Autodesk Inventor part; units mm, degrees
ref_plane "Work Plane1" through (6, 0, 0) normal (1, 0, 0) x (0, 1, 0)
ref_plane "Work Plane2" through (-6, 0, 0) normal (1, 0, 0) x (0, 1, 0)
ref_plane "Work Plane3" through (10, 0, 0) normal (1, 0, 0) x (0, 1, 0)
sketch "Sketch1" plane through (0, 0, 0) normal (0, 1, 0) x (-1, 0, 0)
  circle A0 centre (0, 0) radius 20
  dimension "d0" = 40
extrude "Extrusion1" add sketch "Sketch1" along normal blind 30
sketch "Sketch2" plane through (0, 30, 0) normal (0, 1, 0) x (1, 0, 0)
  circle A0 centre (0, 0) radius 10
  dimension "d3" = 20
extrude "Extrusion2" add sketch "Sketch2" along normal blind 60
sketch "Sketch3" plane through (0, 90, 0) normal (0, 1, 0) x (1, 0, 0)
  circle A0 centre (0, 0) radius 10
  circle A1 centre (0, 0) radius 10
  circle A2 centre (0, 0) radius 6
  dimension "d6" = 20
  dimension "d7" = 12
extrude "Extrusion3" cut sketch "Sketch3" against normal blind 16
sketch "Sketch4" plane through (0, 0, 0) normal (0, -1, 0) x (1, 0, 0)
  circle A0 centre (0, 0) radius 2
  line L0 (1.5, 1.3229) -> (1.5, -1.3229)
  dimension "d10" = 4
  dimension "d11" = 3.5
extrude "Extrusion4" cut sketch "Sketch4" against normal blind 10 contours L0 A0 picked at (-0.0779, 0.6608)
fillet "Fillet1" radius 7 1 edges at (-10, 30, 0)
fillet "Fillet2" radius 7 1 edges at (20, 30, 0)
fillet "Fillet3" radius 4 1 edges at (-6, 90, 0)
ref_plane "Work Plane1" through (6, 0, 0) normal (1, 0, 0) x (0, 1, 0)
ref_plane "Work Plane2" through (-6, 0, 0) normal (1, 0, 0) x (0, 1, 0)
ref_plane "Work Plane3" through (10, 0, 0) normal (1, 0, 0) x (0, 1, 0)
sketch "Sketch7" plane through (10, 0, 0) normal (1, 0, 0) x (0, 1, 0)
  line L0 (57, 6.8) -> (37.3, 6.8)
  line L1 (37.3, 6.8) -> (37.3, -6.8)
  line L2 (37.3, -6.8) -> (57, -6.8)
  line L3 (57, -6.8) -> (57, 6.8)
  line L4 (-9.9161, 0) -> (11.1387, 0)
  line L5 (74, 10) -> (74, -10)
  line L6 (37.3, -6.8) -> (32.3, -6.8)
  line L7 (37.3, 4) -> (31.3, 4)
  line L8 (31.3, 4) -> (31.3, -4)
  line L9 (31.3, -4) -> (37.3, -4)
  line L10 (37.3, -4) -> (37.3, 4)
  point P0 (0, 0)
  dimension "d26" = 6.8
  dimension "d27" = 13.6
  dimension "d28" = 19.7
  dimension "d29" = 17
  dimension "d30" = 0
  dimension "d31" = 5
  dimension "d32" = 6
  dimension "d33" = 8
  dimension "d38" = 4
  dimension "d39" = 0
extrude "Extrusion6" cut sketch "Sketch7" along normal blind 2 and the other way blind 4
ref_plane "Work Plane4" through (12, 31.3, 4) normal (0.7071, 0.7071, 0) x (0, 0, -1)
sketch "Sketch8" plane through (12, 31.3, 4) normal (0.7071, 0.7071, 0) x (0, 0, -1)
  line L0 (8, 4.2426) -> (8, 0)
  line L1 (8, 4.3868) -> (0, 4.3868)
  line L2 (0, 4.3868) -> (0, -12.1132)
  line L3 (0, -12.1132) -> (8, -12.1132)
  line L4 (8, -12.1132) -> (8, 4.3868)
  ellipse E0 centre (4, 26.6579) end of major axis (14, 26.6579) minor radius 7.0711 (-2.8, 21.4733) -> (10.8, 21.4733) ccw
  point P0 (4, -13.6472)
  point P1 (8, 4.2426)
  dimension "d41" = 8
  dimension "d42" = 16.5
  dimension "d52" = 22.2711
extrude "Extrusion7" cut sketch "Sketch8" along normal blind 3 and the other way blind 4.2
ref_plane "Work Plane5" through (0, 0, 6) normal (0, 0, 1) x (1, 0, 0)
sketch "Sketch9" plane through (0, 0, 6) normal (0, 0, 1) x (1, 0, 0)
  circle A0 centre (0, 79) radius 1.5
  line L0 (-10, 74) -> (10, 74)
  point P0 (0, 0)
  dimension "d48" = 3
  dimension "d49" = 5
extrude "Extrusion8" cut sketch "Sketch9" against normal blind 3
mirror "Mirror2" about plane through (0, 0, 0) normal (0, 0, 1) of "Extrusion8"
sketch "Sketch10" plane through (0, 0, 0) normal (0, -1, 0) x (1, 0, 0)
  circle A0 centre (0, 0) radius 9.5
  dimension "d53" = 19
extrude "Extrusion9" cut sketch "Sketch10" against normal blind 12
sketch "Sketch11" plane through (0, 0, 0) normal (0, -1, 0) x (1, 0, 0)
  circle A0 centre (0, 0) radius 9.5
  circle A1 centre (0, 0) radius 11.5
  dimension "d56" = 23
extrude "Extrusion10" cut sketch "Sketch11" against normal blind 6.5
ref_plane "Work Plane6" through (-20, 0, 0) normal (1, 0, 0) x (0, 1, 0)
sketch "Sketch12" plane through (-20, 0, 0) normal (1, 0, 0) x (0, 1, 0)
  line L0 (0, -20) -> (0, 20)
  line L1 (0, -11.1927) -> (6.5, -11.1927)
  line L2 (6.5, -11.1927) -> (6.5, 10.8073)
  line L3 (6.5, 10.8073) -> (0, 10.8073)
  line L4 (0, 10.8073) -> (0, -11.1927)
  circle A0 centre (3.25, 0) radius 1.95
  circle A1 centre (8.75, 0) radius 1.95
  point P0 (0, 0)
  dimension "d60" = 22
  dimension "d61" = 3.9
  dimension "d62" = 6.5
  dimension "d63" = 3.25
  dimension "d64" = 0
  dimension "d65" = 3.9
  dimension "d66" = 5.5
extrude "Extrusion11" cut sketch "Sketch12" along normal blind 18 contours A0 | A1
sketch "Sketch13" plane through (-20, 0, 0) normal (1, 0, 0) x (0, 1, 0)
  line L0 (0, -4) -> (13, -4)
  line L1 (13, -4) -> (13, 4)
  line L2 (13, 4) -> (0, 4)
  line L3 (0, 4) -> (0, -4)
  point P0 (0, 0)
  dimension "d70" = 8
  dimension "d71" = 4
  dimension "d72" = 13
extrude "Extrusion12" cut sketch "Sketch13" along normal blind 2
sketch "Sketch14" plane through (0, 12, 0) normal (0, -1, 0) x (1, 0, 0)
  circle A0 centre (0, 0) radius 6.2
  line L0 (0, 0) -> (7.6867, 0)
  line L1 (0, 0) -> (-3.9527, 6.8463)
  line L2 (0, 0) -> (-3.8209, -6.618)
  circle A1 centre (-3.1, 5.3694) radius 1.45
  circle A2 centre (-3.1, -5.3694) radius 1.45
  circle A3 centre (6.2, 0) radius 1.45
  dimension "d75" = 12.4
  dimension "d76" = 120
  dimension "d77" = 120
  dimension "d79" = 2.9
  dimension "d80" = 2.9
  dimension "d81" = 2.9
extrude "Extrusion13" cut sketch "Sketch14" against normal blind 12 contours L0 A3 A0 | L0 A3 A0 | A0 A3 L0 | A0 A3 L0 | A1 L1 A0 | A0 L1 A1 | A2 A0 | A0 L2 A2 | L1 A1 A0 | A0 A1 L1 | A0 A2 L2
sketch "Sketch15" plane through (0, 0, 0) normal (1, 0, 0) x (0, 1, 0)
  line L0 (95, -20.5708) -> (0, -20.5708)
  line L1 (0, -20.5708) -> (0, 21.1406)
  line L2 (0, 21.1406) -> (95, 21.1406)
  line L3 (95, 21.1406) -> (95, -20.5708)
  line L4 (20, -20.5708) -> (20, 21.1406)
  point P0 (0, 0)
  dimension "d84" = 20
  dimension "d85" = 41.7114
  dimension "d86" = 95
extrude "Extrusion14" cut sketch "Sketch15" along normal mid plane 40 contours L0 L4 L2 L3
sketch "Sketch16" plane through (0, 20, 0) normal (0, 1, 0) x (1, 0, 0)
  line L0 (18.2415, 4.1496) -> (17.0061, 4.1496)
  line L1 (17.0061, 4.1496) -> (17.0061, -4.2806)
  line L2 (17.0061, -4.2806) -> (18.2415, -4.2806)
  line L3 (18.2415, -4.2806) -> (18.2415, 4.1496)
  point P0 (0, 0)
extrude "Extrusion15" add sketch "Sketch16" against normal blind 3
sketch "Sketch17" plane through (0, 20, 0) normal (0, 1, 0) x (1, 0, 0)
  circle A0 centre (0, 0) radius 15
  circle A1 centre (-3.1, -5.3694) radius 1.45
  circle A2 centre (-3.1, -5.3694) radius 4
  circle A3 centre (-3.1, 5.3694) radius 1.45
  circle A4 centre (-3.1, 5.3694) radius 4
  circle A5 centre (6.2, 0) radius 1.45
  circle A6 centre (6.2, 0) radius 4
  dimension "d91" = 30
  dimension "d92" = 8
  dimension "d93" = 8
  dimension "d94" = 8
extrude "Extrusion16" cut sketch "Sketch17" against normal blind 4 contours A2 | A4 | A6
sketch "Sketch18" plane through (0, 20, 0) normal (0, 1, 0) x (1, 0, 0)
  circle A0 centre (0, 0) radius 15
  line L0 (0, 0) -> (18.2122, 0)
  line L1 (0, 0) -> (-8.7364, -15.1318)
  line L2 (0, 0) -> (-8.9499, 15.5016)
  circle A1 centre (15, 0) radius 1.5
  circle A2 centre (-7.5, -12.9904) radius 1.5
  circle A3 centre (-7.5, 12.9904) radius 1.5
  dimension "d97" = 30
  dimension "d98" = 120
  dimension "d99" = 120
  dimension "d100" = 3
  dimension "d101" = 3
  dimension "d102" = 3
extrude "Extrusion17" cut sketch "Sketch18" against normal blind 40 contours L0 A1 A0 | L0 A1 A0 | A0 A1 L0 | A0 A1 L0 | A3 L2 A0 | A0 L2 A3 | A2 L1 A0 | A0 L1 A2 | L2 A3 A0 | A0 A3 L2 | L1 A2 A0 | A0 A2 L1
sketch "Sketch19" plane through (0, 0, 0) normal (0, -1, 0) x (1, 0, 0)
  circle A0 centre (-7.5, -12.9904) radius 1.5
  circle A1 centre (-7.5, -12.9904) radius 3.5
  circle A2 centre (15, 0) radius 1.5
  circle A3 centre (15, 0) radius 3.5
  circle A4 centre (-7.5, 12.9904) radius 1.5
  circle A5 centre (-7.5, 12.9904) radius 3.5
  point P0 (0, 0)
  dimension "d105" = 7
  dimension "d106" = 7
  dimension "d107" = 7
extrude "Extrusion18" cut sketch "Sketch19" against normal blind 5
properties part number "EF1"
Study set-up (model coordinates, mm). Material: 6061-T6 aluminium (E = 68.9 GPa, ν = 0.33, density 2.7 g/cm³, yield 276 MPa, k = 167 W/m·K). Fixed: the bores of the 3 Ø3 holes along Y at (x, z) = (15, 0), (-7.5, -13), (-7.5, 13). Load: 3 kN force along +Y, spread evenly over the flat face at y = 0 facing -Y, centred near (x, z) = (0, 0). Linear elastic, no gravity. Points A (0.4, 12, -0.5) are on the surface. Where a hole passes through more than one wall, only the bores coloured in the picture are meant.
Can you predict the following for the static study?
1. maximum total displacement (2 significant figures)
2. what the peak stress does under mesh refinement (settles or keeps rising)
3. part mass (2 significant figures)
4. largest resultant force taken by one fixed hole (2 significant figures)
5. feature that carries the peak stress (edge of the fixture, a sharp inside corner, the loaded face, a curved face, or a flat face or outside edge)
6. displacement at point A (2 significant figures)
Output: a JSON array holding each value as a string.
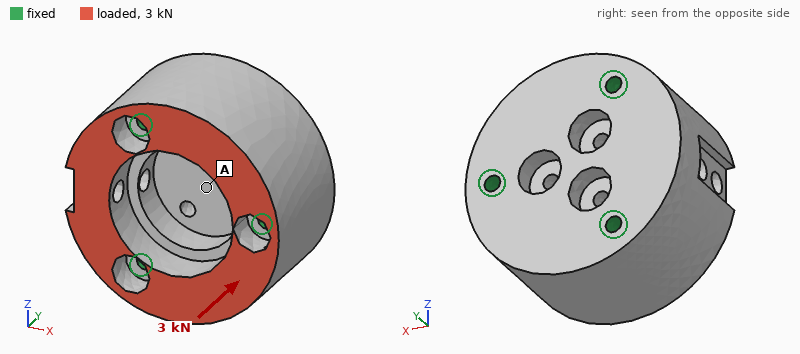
["3.3 µm", "keeps rising", "51 g", "1.0 kN", "a sharp inside corner", "0.53 µm"]
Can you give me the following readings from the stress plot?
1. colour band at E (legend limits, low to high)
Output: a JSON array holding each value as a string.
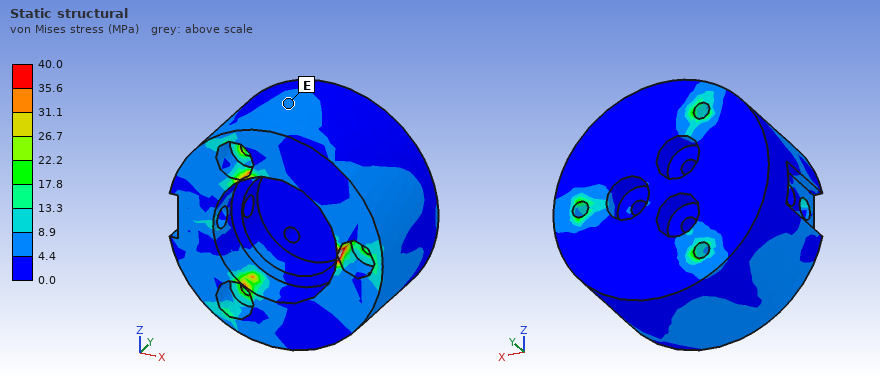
["4.4 to 8.9 MPa"]
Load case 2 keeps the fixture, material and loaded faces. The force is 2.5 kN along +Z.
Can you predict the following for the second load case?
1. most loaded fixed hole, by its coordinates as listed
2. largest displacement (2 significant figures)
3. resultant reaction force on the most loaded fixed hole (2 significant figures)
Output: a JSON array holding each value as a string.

["(15, 0)", "6.8 µm", "1.2 kN"]
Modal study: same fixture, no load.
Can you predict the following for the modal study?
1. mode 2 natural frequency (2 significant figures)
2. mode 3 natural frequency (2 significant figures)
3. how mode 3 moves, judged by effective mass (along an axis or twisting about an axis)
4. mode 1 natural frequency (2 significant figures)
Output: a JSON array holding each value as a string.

["29 kHz", "34 kHz", "along Y", "28 kHz"]
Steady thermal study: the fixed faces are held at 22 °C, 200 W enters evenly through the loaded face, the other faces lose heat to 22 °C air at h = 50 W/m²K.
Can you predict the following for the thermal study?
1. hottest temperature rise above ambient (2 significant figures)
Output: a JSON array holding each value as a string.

["28 K"]
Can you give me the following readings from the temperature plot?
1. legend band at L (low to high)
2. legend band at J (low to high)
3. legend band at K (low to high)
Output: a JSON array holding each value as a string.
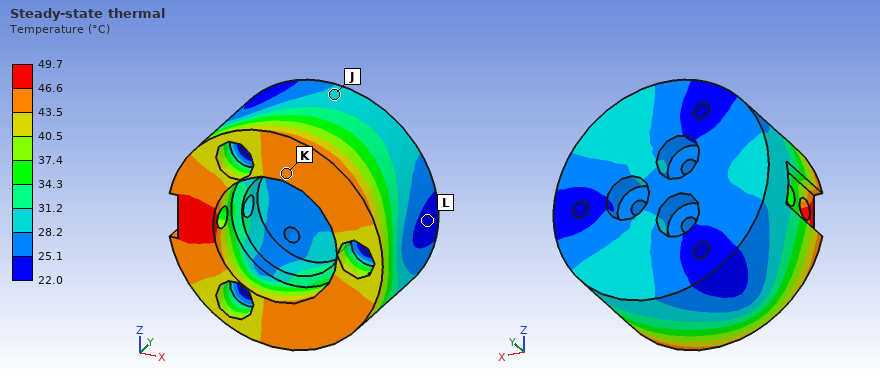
["22.0 to 25.1 °C", "28.2 to 31.2 °C", "43.5 to 46.6 °C"]
